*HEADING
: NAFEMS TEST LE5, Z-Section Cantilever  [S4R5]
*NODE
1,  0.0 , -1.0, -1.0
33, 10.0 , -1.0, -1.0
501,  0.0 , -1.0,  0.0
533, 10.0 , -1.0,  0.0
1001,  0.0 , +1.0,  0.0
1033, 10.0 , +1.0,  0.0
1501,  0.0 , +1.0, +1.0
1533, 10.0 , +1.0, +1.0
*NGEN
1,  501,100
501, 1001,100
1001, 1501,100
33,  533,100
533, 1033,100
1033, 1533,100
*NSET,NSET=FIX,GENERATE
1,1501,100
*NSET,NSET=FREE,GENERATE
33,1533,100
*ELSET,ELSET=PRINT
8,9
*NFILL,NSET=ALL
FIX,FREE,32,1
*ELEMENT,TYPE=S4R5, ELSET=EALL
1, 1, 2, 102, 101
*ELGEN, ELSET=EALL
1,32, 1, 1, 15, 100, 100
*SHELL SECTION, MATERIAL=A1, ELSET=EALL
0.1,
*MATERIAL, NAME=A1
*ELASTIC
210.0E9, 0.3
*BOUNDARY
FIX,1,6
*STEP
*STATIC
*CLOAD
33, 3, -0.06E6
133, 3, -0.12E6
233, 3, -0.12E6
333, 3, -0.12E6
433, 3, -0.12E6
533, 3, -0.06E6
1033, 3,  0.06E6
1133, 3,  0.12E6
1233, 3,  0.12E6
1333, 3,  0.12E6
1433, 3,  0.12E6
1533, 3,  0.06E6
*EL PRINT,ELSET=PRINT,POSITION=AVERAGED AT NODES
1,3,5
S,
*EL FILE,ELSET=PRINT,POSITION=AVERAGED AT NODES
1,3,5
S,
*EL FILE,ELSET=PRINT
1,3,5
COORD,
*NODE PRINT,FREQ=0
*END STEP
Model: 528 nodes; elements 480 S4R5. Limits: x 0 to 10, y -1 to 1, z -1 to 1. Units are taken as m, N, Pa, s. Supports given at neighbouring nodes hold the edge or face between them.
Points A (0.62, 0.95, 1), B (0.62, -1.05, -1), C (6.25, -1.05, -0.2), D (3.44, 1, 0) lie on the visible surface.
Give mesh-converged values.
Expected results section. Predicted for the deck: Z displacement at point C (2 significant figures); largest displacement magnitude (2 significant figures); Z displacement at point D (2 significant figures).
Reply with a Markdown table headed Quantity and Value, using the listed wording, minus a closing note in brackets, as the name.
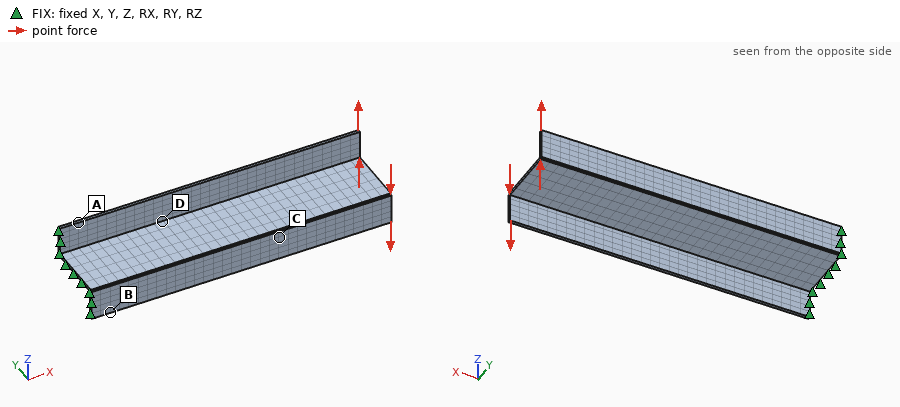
| Quantity | Value |
|---|---|
| Z displacement at point C | -0.016 m |
| largest displacement magnitude | 0.044 m |
| Z displacement at point D | 0.0054 m |
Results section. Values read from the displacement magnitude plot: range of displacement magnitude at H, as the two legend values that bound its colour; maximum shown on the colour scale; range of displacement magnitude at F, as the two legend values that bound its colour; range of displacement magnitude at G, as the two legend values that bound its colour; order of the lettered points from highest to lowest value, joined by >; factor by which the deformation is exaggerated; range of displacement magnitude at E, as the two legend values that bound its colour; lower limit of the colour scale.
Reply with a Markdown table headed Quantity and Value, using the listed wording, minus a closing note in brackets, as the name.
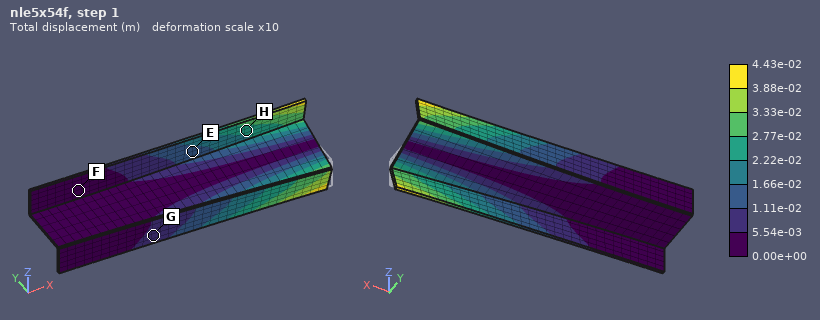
| Quantity | Value |
|---|---|
| range of displacement magnitude at H, as the two legend values that bound its colour | 2.22e-02 to 2.77e-02 m |
| maximum shown on the colour scale | 4.43e-02 m |
| range of displacement magnitude at F, as the two legend values that bound its colour | 0.00e+00 to 5.54e-03 m |
| range of displacement magnitude at G, as the two legend values that bound its colour | 5.54e-03 to 1.11e-02 m |
| order of the lettered points from highest to lowest value, joined by > | H > E > G > F |
| factor by which the deformation is exaggerated | 10 |
| range of displacement magnitude at E, as the two legend values that bound its colour | 1.11e-02 to 1.66e-02 m |
| lower limit of the colour scale | 0.00e+00 m |
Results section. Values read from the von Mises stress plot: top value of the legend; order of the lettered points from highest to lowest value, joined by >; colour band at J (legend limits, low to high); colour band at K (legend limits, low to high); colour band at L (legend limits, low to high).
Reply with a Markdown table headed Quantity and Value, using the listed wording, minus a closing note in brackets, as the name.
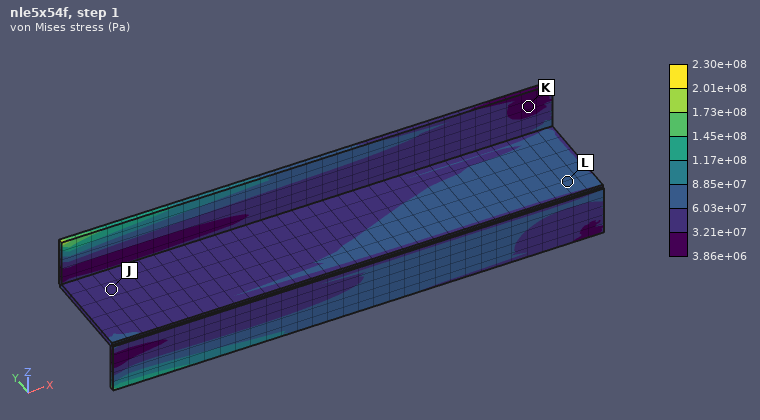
| Quantity | Value |
|---|---|
| top value of the legend | 2.30e+08 Pa |
| order of the lettered points from highest to lowest value, joined by > | L > J > K |
| colour band at J | 3.21e+07 to 6.03e+07 Pa |
| colour band at K | 3.86e+06 to 3.21e+07 Pa |
| colour band at L | 6.03e+07 to 8.85e+07 Pa |
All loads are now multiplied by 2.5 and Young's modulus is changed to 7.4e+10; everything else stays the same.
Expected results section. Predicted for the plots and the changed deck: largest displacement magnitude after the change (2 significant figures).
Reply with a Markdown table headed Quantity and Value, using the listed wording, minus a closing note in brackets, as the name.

| Quantity | Value |
|---|---|
| largest displacement magnitude after the change | 0.31 m |
